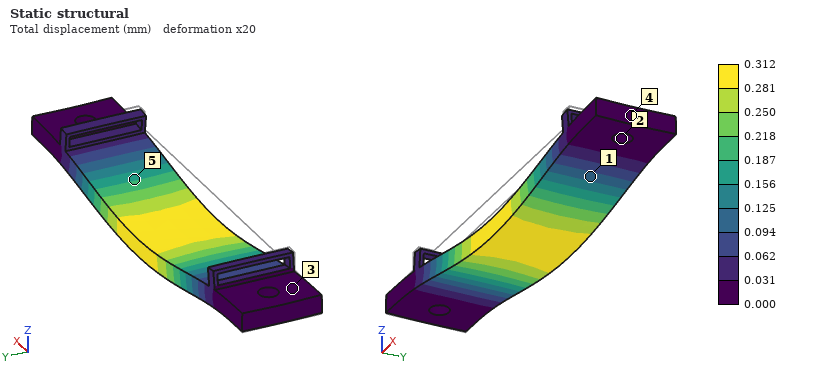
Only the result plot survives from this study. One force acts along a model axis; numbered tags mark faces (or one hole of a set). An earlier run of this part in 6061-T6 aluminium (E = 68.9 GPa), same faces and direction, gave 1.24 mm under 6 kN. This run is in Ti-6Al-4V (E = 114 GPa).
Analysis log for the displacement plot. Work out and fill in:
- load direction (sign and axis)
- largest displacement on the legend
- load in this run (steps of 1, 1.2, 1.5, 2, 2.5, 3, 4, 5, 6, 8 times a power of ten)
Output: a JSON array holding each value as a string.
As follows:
["-Z", "0.312 mm", "2.5 kN"]
